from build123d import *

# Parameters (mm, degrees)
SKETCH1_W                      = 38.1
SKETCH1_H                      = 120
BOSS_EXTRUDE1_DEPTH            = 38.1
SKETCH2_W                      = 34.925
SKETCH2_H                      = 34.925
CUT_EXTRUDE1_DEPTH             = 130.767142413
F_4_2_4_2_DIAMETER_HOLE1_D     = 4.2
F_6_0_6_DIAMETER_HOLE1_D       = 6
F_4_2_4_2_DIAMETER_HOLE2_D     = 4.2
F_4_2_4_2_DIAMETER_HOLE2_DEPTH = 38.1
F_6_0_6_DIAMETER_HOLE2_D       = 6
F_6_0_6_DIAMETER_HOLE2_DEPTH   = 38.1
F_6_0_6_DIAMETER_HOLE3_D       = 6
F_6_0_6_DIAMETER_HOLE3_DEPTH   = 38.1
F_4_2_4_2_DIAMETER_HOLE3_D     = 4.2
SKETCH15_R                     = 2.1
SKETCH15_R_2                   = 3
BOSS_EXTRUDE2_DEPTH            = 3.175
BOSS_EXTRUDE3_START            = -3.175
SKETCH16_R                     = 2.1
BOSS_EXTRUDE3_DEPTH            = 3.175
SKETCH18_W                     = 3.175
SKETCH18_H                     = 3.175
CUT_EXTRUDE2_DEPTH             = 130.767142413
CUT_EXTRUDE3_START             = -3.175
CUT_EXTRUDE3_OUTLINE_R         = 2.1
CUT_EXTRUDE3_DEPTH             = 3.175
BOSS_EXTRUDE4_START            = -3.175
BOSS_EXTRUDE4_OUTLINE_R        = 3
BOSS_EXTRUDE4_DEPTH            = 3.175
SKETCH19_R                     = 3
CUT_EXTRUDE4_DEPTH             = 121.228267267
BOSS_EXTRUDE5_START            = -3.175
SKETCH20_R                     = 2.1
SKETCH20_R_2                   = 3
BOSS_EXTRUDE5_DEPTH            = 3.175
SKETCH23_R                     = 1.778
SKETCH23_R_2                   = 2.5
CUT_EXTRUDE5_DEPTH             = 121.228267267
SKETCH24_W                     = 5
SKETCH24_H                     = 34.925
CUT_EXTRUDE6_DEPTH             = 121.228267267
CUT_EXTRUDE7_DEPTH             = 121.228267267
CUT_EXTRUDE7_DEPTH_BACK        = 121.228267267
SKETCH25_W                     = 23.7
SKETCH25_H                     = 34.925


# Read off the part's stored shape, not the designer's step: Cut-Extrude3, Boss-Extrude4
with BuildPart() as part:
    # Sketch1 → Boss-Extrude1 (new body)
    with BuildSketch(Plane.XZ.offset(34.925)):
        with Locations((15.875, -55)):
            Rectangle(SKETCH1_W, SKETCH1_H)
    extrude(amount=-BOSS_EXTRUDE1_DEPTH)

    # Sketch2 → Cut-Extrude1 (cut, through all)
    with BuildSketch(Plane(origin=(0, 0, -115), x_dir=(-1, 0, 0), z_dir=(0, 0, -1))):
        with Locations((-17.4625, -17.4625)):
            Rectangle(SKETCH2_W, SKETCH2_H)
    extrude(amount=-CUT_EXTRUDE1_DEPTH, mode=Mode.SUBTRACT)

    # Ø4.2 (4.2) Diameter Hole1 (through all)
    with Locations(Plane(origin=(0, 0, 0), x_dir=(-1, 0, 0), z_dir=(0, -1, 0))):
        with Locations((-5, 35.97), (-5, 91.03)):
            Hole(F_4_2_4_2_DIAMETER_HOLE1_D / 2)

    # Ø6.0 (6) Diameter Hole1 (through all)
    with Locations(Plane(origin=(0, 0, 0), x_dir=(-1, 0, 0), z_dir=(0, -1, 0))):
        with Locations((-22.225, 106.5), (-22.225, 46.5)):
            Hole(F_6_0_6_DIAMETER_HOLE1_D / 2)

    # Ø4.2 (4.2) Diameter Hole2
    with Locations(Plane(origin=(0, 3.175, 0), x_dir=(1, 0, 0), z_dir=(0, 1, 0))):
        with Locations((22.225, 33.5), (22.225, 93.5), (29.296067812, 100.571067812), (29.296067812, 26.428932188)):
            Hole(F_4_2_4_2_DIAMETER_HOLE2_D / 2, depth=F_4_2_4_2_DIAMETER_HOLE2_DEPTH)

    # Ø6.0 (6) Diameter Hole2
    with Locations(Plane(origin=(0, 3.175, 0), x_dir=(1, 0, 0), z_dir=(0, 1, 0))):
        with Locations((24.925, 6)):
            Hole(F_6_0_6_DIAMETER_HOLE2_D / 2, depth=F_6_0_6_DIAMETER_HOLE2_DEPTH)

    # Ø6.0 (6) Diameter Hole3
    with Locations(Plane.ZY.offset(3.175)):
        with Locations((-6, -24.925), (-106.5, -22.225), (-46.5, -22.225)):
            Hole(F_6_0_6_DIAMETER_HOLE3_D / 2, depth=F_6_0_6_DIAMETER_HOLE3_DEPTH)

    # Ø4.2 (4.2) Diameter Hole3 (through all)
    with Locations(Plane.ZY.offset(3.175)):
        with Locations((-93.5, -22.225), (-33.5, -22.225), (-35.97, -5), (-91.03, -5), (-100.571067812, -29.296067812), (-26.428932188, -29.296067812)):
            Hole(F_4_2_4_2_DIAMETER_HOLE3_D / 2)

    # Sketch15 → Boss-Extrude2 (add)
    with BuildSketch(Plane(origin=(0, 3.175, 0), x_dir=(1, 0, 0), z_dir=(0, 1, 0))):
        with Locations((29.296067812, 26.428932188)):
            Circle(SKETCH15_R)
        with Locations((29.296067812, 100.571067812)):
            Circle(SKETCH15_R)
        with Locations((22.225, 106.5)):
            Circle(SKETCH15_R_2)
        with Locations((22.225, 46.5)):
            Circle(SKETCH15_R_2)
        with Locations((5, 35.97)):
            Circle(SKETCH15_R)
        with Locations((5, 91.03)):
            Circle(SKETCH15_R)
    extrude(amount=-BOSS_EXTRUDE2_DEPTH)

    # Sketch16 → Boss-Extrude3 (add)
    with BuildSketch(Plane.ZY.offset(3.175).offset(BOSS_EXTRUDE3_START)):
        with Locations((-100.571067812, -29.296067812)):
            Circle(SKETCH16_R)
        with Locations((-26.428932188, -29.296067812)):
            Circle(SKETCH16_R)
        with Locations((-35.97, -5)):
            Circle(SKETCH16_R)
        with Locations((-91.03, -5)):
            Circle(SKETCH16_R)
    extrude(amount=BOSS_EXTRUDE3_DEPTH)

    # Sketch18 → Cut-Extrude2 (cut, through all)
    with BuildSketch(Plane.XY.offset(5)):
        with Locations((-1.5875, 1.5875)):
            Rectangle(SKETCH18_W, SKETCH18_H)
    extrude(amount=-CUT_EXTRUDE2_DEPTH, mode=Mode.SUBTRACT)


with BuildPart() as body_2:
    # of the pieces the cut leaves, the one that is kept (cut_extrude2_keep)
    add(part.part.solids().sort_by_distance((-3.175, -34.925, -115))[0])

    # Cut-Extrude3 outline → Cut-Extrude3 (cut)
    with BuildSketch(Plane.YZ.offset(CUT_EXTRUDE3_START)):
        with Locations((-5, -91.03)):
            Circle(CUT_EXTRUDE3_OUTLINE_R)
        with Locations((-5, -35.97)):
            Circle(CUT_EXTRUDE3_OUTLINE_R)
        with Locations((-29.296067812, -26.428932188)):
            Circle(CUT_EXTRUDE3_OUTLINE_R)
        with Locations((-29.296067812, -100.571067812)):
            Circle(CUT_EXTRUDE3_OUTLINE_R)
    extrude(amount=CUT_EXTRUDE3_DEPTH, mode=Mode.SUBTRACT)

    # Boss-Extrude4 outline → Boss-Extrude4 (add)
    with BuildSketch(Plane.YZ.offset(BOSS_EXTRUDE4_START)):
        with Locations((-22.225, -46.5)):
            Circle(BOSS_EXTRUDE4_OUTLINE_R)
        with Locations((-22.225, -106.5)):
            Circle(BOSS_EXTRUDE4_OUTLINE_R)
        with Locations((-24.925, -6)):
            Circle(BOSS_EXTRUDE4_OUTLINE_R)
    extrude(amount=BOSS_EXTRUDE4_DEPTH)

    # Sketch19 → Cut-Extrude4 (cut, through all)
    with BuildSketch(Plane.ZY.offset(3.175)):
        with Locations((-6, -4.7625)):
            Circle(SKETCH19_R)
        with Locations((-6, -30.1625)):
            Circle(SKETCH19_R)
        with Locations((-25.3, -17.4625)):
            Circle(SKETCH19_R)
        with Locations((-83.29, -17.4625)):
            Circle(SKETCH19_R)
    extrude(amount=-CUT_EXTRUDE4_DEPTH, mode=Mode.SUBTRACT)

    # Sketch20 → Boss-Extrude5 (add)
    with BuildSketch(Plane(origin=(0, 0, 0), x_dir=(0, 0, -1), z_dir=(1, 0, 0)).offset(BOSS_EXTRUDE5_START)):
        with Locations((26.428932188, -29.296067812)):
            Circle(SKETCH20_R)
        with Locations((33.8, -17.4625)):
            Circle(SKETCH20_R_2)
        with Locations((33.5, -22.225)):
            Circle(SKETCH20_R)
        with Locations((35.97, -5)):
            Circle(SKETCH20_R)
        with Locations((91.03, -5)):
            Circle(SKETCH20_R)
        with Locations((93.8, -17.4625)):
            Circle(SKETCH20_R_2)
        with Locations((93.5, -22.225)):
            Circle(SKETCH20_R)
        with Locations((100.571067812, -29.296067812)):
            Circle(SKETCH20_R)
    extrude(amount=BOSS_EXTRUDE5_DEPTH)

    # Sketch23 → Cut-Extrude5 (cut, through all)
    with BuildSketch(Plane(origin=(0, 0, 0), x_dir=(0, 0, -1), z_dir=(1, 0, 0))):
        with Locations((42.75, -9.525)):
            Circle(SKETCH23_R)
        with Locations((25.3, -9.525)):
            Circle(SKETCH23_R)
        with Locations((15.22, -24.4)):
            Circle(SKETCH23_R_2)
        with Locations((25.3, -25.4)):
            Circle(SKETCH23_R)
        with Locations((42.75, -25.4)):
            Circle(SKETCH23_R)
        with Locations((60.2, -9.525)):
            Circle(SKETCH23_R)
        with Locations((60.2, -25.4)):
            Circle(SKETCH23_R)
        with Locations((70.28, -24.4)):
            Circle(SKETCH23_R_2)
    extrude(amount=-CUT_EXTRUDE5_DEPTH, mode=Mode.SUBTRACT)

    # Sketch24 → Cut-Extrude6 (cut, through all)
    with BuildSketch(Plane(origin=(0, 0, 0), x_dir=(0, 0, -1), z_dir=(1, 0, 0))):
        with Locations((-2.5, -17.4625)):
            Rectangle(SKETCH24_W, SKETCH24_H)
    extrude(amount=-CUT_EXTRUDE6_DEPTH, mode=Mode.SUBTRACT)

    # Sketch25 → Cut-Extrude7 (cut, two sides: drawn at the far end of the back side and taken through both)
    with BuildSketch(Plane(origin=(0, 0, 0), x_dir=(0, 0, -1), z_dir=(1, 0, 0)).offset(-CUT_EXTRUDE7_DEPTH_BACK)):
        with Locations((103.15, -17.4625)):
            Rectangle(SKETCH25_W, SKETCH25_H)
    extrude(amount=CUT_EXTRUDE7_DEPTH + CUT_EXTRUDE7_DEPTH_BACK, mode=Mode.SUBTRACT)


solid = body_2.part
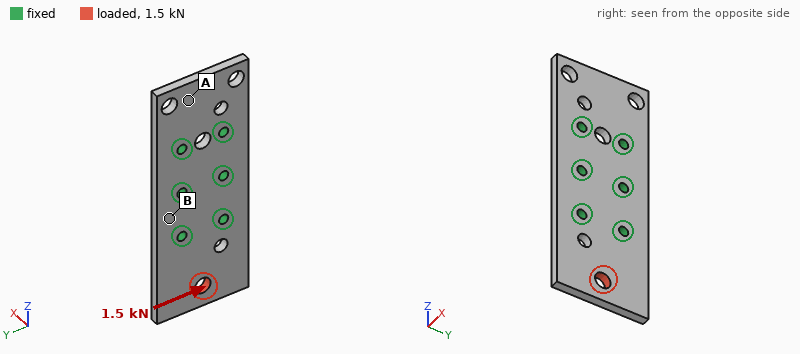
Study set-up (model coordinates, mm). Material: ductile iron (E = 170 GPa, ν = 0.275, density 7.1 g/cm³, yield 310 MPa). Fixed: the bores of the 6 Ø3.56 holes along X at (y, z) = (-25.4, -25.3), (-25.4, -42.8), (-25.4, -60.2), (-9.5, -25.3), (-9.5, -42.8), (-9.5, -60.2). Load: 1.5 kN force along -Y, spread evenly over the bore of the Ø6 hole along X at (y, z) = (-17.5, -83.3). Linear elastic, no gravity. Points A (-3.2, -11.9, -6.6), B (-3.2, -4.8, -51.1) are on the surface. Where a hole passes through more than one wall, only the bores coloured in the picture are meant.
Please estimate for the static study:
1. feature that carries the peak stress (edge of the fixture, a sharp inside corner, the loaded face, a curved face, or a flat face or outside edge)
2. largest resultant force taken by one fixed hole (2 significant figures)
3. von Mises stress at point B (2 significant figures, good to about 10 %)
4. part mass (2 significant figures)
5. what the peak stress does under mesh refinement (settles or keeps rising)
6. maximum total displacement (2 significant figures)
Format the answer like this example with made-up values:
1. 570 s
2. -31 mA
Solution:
1. edge of the fixture
2. 1.5 kN
3. 16 MPa
4. 67 g
5. keeps rising
6. 17 µm
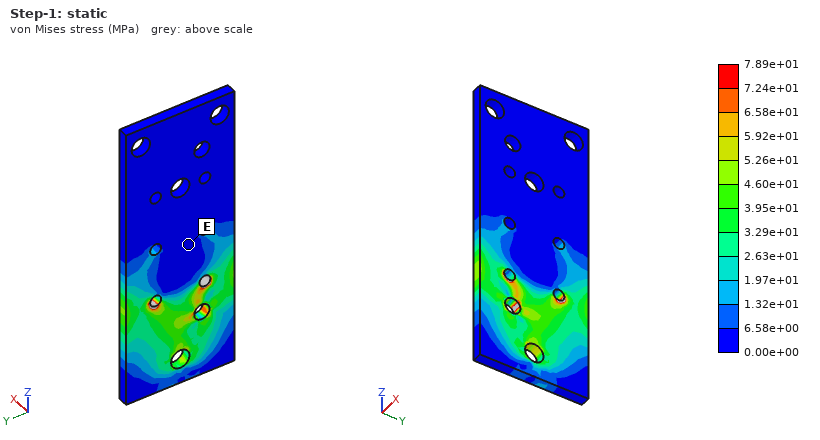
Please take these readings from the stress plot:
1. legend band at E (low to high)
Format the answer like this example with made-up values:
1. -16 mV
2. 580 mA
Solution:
1. 0.00e+00 to 6.58e+00 MPa
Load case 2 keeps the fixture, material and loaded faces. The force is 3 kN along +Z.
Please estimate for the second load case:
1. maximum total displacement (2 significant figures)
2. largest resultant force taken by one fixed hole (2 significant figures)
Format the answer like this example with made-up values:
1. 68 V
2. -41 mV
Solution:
1. 8.9 µm
2. 1.3 kN
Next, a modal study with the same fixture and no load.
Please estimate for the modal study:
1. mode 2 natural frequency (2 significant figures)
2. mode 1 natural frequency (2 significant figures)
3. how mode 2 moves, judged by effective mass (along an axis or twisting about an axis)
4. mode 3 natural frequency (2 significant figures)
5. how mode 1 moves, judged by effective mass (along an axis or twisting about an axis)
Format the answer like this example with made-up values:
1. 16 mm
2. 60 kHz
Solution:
1. 4000 Hz
2. 2600 Hz
3. along X
4. 5300 Hz
5. along X
